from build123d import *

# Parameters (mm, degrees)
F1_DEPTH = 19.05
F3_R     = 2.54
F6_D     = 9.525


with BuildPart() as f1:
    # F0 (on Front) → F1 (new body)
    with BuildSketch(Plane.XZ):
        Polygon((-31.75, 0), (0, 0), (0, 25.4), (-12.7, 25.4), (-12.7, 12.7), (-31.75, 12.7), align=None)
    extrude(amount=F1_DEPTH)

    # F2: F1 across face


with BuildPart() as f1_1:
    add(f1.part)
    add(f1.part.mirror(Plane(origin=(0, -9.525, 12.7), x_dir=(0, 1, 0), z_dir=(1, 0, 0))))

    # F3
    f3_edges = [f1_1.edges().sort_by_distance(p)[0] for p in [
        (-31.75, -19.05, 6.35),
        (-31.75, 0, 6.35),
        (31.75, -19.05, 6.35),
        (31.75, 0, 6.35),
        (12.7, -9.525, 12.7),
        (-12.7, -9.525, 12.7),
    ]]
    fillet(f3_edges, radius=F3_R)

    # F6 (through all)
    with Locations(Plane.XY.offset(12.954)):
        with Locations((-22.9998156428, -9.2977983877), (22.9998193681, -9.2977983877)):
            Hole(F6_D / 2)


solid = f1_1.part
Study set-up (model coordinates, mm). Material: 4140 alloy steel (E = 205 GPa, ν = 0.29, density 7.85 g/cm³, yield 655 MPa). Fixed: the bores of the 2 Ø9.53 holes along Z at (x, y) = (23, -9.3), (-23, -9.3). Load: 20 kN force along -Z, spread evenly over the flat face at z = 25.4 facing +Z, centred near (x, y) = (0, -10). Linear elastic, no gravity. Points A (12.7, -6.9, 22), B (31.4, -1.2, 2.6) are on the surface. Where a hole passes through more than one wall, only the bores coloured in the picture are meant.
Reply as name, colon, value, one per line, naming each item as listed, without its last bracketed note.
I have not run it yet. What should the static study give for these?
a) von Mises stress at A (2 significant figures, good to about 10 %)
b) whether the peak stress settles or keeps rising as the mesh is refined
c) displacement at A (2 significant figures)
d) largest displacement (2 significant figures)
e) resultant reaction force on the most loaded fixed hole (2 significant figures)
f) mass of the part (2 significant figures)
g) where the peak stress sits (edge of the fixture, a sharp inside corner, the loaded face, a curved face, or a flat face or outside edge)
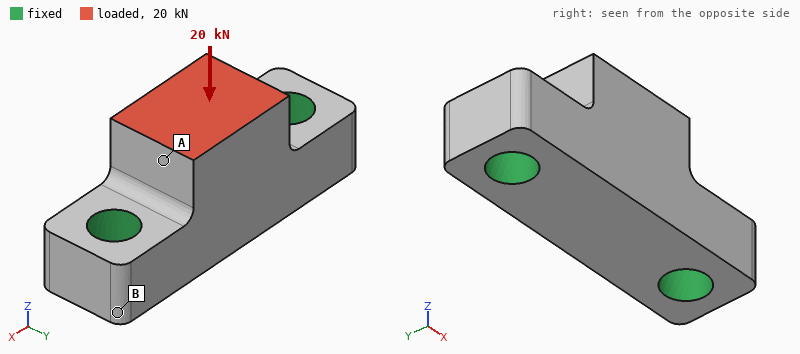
von Mises stress at A: 44 MPa
whether the peak stress settles or keeps rising as the mesh is refined: keeps rising
displacement at A: 10 µm
largest displacement: 11 µm
resultant reaction force on the most loaded fixed hole: 11 kN
mass of the part: 150 g
where the peak stress sits: edge of the fixture
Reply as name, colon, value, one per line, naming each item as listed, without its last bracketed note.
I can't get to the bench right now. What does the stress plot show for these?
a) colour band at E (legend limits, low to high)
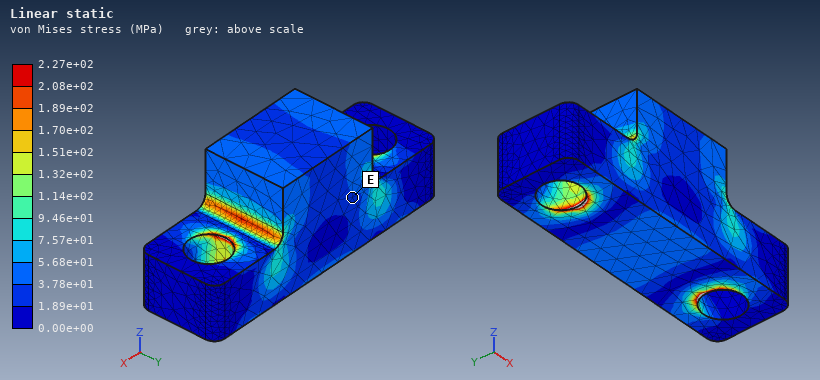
colour band at E: 1.89e+01 to 3.78e+01 MPa
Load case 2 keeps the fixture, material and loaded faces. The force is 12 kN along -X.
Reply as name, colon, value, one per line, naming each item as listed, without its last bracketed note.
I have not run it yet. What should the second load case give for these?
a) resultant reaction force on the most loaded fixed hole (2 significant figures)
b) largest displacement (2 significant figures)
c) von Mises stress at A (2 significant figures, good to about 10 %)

resultant reaction force on the most loaded fixed hole: 8.7 kN
largest displacement: 15 µm
von Mises stress at A: 38 MPa
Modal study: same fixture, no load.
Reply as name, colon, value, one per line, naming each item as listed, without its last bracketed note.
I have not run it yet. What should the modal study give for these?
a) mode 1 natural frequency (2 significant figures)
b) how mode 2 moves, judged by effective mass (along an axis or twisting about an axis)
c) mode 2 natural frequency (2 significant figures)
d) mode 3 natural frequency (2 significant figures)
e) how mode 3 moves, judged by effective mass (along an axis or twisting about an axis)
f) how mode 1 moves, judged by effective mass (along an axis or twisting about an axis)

mode 1 natural frequency: 14 kHz
how mode 2 moves, judged by effective mass: along Z
mode 2 natural frequency: 24 kHz
mode 3 natural frequency: 29 kHz
how mode 3 moves, judged by effective mass: along Y
how mode 1 moves, judged by effective mass: along Y
